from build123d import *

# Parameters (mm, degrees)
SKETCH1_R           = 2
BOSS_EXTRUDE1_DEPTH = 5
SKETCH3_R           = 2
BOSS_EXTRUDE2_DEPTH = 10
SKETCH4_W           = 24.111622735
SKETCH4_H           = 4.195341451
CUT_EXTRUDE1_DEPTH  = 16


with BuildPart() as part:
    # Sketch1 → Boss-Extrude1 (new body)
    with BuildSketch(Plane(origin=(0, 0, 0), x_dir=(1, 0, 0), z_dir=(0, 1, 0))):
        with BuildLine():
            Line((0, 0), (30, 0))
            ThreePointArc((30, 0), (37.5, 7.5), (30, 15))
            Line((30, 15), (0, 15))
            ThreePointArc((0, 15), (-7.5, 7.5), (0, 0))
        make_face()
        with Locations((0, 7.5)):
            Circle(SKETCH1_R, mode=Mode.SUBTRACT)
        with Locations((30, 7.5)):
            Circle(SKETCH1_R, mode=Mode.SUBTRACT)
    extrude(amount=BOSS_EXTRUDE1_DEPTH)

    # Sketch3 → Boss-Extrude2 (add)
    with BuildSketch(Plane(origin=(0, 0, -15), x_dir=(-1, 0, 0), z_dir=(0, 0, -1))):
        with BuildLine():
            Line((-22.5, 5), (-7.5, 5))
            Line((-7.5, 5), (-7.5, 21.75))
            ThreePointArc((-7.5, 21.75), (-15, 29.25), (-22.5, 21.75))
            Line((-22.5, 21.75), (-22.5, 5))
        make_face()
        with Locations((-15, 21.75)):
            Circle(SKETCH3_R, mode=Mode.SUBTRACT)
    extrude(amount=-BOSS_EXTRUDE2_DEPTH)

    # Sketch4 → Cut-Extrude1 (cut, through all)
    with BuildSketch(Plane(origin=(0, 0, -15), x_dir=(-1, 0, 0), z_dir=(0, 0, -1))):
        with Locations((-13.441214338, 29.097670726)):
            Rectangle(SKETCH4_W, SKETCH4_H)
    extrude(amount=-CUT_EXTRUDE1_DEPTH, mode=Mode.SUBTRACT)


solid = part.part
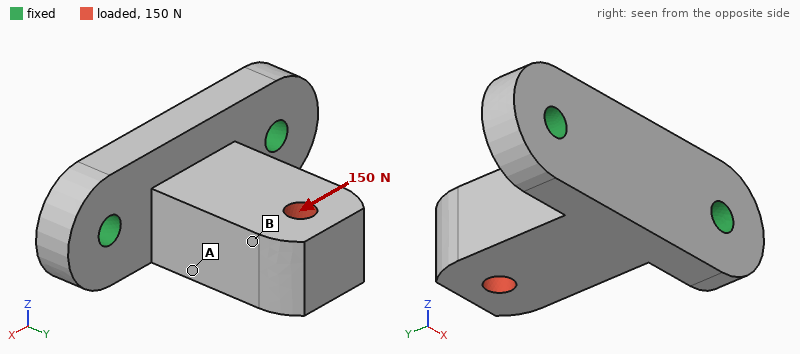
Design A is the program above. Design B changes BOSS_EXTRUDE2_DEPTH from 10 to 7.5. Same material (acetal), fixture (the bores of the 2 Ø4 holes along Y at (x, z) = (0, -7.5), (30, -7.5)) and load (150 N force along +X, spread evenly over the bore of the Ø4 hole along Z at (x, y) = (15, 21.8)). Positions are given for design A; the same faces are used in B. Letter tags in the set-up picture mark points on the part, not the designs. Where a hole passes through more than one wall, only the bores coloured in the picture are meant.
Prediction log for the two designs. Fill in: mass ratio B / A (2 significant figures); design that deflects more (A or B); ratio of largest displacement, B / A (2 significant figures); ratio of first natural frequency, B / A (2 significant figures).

0.87
B
1.3
1.0
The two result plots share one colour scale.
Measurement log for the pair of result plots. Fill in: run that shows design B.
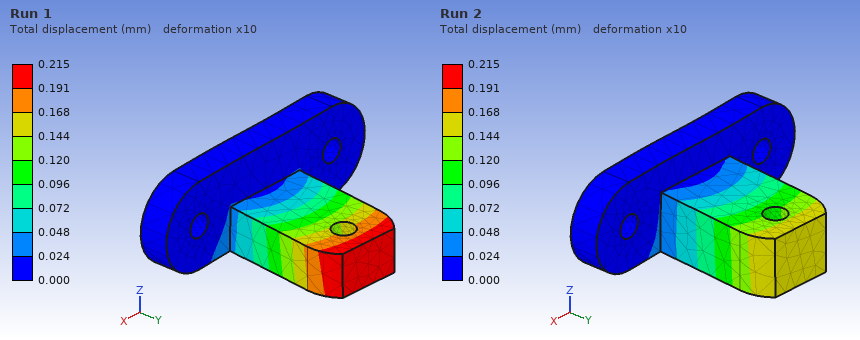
Run 1
